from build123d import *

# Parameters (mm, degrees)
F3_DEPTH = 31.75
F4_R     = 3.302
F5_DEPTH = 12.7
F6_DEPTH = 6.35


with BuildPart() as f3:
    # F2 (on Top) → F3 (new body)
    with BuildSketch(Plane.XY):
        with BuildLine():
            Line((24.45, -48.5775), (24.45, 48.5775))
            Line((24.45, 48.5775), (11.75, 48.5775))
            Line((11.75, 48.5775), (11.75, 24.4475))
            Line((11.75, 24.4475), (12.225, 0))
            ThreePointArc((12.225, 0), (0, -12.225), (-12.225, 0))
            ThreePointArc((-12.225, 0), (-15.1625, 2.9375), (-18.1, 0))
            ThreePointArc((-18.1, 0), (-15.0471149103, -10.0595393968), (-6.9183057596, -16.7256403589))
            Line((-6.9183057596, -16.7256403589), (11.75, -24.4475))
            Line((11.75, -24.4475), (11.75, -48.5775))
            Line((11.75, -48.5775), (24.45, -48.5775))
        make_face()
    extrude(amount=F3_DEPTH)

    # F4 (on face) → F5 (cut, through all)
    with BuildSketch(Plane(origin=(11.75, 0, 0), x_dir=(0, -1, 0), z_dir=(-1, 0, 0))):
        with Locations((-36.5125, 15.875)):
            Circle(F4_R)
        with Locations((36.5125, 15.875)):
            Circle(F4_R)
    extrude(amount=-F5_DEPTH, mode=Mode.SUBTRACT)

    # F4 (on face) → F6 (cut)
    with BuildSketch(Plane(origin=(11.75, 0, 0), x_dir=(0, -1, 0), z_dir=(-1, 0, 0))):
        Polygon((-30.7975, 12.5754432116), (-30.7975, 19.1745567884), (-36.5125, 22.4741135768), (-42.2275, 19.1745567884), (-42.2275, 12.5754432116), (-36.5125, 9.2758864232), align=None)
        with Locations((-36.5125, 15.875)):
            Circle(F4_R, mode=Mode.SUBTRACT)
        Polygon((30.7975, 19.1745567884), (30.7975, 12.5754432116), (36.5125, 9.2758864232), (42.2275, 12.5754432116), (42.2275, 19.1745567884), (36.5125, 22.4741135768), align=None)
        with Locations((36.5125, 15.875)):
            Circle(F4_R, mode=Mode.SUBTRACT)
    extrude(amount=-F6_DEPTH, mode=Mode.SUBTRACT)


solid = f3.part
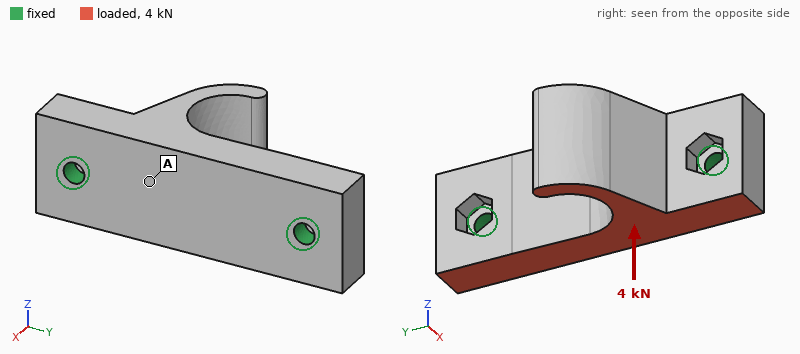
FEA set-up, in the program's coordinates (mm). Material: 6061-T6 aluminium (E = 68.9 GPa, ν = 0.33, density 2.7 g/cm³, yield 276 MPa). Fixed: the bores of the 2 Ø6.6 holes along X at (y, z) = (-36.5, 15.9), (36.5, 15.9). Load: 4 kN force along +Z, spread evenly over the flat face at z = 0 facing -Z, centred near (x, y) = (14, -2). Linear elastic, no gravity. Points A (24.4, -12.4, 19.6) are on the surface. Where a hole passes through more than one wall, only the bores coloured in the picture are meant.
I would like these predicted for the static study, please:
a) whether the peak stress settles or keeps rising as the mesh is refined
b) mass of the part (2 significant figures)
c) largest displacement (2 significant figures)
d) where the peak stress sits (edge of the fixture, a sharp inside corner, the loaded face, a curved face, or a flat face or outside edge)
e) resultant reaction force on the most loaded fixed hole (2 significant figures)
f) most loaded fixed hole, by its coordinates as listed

keeps rising
130 g
70 µm
edge of the fixture
2.1 kN
(-36.5, 15.9)
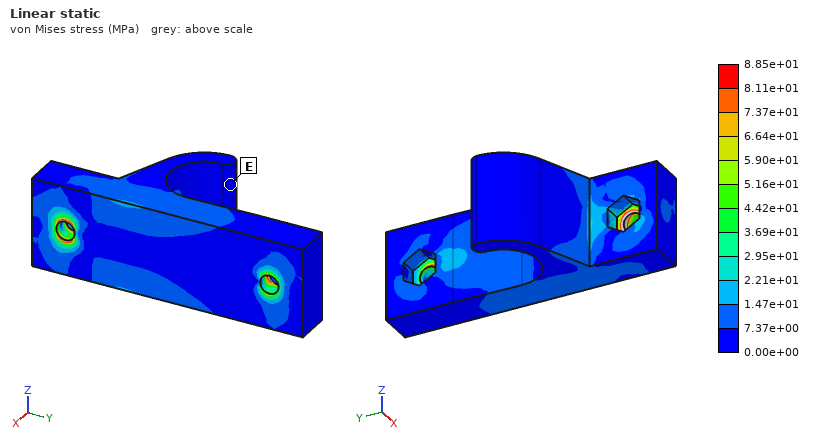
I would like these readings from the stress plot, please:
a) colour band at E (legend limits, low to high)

0.00e+00 to 7.37e+00 MPa
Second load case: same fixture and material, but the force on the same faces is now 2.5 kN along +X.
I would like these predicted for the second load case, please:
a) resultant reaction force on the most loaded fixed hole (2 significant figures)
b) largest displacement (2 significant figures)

1.5 kN
88 µm
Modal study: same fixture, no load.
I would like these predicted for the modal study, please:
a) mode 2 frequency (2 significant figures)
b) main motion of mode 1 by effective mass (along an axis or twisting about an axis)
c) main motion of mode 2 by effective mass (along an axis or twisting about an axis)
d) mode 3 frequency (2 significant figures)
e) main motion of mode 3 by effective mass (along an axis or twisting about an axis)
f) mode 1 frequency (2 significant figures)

4900 Hz
along Z
along X
8300 Hz
along X
4200 Hz
